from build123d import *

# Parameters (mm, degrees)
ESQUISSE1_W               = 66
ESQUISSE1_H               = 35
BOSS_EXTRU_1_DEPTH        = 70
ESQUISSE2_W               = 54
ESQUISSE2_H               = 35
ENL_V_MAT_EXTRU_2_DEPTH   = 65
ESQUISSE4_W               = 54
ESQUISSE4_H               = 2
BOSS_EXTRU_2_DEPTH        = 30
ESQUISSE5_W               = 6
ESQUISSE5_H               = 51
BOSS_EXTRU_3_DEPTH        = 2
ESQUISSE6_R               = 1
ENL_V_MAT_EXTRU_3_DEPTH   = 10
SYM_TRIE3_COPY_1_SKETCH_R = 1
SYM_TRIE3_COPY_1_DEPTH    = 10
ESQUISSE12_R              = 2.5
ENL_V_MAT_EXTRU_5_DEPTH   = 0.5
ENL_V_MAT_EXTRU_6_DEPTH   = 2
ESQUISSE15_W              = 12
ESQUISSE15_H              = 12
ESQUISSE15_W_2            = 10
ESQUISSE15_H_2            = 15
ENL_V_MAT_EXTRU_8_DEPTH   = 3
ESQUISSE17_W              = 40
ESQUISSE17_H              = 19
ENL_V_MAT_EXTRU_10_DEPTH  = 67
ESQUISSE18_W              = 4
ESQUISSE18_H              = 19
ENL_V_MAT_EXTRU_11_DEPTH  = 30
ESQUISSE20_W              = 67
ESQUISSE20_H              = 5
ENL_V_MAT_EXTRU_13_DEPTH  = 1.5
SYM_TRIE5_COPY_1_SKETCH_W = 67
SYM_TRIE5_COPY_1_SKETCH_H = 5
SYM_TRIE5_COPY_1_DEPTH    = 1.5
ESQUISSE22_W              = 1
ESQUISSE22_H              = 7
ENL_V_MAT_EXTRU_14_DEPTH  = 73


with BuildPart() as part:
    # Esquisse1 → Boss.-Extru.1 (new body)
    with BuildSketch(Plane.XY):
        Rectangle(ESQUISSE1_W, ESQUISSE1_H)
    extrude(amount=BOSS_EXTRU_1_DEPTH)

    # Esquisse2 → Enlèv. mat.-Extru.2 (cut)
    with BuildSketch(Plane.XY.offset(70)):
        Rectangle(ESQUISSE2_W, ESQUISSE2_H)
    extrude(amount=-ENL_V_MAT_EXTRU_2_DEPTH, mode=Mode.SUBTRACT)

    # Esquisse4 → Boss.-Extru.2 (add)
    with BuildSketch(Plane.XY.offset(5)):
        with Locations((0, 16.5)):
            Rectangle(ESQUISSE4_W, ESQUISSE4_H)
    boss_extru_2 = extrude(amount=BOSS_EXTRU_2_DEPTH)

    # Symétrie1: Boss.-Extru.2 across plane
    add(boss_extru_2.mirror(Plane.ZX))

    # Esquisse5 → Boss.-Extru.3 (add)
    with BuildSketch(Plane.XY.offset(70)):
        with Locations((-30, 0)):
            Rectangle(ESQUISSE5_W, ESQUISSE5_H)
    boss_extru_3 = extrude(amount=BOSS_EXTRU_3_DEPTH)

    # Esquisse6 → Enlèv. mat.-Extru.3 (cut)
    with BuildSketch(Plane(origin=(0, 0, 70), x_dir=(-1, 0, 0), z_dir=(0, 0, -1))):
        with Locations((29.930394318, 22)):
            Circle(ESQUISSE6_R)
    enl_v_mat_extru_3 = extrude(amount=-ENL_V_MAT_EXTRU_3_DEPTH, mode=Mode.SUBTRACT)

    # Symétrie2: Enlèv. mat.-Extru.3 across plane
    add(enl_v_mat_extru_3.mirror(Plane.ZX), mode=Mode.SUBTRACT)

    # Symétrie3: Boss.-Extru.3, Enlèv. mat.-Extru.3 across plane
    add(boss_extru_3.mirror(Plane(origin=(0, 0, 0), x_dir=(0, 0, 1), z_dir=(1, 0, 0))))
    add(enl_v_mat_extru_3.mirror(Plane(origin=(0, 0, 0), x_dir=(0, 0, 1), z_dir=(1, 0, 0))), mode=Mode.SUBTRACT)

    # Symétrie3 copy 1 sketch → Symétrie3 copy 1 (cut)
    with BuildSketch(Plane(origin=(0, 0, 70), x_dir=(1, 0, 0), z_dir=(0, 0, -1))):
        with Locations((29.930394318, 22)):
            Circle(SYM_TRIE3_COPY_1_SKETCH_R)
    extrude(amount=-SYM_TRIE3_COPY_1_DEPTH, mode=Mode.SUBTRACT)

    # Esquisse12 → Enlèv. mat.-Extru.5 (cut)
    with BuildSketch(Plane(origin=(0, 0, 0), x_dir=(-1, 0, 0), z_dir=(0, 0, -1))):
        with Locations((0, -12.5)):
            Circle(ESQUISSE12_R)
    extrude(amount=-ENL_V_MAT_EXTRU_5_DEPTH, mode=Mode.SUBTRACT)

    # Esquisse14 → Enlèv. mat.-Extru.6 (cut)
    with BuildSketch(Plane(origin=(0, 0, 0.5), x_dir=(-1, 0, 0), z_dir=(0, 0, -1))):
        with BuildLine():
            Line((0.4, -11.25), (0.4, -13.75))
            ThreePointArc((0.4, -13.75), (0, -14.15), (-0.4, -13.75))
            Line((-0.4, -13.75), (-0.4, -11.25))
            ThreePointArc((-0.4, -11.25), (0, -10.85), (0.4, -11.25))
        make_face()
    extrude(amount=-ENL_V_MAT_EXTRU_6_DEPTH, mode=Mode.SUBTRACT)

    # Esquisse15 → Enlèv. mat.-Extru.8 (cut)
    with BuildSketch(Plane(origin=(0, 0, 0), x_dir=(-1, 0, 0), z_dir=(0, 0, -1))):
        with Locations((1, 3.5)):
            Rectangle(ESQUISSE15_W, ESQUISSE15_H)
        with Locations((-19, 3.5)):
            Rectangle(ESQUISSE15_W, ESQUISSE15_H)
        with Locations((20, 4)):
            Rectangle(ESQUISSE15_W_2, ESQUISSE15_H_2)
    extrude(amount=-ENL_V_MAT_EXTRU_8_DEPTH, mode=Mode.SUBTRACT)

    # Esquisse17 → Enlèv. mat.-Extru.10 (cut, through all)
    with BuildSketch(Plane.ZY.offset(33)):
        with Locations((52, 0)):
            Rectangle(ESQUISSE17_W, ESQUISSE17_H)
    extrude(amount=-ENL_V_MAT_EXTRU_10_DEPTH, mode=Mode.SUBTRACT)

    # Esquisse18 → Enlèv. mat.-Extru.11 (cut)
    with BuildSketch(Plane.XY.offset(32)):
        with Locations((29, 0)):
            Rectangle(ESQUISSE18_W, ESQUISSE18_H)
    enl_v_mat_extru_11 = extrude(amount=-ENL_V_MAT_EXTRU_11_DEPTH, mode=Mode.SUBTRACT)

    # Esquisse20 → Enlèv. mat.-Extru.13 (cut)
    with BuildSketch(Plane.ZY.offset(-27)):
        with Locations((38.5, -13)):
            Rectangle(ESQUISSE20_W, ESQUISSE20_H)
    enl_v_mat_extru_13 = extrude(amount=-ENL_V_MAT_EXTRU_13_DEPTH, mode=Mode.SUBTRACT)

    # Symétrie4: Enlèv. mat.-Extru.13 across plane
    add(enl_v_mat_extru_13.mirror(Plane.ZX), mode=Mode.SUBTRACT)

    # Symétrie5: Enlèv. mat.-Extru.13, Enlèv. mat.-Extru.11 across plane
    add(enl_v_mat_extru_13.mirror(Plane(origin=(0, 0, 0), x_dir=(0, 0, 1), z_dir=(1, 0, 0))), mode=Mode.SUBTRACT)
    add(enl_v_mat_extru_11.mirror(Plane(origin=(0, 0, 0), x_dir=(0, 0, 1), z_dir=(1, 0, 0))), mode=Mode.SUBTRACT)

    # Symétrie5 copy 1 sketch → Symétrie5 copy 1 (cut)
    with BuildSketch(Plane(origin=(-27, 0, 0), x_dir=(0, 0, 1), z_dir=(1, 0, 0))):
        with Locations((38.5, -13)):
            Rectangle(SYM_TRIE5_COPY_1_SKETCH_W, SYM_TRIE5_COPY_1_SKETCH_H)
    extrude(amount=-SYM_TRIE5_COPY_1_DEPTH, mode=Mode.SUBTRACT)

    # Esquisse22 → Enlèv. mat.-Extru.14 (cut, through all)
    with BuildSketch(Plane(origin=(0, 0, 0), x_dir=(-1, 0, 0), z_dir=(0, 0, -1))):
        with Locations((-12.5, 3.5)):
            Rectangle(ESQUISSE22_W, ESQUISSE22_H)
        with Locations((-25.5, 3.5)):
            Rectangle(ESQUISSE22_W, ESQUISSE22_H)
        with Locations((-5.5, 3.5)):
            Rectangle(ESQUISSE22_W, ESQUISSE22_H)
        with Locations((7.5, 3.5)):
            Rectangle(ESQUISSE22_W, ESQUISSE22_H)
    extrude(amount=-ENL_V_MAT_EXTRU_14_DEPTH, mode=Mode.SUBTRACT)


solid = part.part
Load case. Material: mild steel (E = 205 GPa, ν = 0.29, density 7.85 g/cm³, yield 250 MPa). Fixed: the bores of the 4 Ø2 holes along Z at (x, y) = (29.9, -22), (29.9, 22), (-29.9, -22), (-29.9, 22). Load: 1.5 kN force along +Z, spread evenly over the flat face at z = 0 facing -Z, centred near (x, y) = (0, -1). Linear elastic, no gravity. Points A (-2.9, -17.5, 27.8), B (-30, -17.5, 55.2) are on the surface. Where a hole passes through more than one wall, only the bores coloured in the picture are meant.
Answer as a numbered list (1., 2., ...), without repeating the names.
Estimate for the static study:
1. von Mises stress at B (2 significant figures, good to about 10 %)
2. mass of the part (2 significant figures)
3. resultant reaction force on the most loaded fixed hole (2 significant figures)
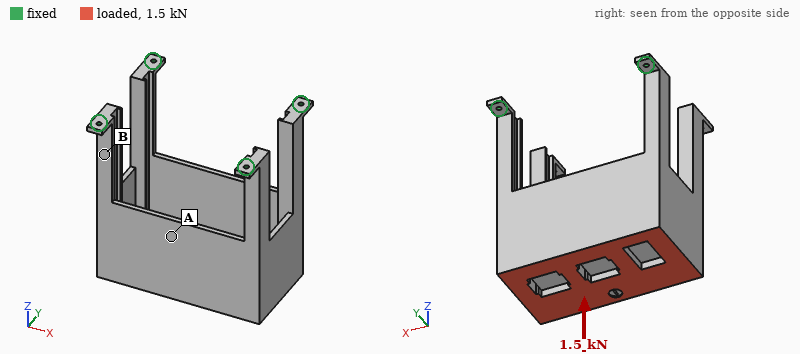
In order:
1. 27 MPa
2. 230 g
3. 400 N
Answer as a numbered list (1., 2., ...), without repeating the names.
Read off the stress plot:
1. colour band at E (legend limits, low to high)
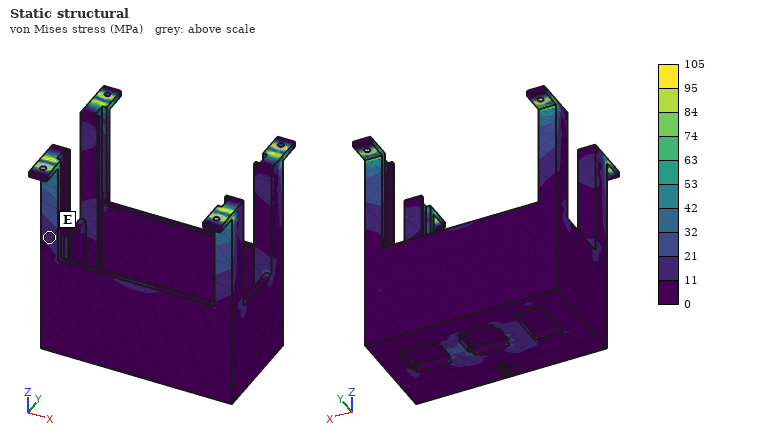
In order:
1. 11 to 21 MPa
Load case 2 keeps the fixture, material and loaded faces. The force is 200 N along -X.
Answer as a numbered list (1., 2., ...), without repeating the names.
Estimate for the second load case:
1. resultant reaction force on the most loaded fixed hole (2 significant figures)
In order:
1. 120 N
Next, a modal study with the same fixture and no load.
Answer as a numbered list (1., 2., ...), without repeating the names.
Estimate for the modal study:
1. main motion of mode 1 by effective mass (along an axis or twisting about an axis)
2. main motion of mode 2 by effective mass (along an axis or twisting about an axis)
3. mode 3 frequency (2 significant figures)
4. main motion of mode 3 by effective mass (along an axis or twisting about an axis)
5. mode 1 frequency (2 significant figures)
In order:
1. along X
2. along Y
3. 1500 Hz
4. twisting about Z
5. 700 Hz
